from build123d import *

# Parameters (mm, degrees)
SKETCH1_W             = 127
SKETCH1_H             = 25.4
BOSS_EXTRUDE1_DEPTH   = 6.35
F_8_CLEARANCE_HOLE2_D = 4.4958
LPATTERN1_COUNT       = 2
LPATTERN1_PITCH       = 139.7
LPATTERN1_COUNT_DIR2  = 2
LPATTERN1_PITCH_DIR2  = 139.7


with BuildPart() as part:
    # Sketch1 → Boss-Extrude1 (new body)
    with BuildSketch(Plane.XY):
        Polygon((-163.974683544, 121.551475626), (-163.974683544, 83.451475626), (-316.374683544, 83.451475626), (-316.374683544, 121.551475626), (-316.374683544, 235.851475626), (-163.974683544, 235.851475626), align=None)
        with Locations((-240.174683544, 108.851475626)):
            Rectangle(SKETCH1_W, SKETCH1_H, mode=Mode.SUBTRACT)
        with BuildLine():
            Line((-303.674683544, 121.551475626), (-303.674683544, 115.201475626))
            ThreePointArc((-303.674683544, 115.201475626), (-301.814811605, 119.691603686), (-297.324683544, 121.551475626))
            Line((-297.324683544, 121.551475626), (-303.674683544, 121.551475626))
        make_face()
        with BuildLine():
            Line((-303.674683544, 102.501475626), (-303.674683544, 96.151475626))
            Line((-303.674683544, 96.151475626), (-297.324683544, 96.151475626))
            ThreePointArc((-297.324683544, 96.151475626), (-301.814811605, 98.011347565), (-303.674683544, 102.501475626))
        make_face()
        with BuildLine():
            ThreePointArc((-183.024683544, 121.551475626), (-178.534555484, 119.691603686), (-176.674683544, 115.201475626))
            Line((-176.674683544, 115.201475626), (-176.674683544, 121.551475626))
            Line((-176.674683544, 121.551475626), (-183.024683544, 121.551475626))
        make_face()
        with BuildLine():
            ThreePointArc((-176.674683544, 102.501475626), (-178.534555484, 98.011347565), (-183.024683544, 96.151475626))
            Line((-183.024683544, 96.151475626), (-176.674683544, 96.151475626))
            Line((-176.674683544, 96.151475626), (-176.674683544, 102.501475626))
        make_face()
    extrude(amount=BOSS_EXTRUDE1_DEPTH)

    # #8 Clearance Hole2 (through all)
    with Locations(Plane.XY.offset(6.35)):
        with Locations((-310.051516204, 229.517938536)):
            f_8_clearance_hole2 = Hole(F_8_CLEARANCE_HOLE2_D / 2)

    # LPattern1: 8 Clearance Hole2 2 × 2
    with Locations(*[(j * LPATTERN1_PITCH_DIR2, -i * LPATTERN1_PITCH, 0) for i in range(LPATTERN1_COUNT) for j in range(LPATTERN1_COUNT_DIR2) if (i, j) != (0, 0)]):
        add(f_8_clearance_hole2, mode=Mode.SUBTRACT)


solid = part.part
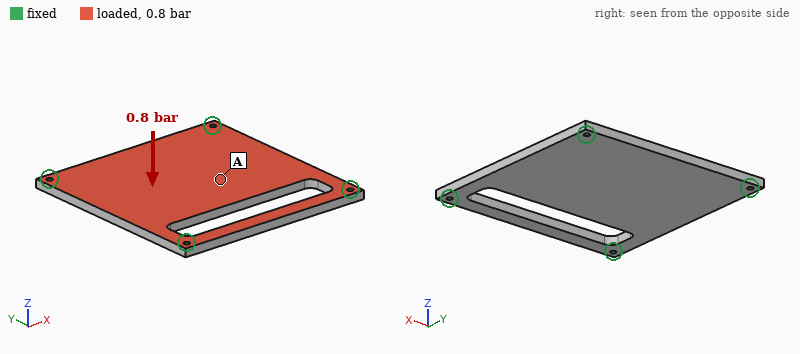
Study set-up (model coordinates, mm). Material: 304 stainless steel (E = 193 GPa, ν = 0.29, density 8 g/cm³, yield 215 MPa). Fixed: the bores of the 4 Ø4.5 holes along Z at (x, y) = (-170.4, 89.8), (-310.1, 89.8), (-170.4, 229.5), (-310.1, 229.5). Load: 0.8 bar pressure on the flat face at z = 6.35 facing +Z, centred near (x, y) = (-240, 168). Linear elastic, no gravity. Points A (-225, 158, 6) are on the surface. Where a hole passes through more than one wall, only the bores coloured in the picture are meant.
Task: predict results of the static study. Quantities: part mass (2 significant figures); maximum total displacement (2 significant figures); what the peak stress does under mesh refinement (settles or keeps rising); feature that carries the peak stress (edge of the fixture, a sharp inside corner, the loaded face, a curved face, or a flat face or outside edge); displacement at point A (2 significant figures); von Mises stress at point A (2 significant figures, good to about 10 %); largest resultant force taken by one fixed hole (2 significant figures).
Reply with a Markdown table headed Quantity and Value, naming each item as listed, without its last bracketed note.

| Quantity | Value |
|---|---|
| part mass | 1.0 kg |
| maximum total displacement | 94 µm |
| what the peak stress does under mesh refinement | keeps rising |
| feature that carries the peak stress | edge of the fixture |
| displacement at point A | 81 µm |
| von Mises stress at point A | 14 MPa |
| largest resultant force taken by one fixed hole | 450 N |
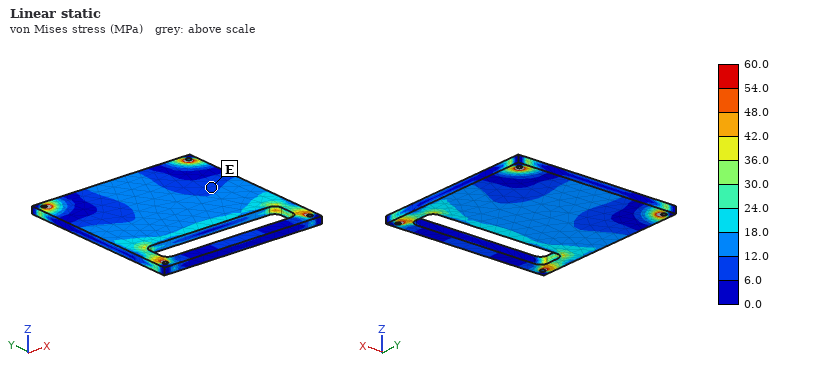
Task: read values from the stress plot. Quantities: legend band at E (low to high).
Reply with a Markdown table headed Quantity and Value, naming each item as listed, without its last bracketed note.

| Quantity | Value |
|---|---|
| legend band at E | 6.0 to 12.0 MPa |
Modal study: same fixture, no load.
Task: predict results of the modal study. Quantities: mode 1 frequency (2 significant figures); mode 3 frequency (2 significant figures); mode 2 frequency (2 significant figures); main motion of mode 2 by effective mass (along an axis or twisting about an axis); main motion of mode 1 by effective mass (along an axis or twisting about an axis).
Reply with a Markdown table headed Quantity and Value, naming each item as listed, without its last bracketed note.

| Quantity | Value |
|---|---|
| mode 1 frequency | 800 Hz |
| mode 3 frequency | 1700 Hz |
| mode 2 frequency | 1600 Hz |
| main motion of mode 2 by effective mass | twisting about Y |
| main motion of mode 1 by effective mass | along Z |
